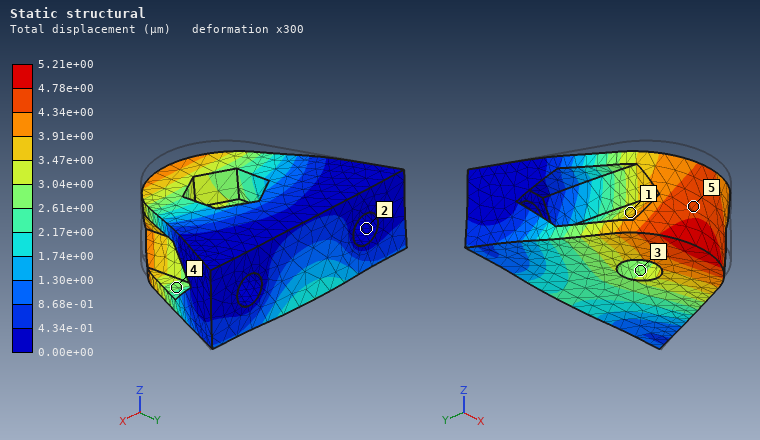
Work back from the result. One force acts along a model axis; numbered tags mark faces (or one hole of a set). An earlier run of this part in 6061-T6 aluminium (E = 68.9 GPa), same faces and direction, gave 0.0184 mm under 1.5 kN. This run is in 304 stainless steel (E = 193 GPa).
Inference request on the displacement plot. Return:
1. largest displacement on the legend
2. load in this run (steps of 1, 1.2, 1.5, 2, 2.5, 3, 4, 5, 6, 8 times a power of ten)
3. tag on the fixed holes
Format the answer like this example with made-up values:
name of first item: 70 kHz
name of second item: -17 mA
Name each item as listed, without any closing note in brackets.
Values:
largest displacement on the legend: 5.21e+00 µm
load in this run: 1.2 kN
tag on the fixed holes: 2
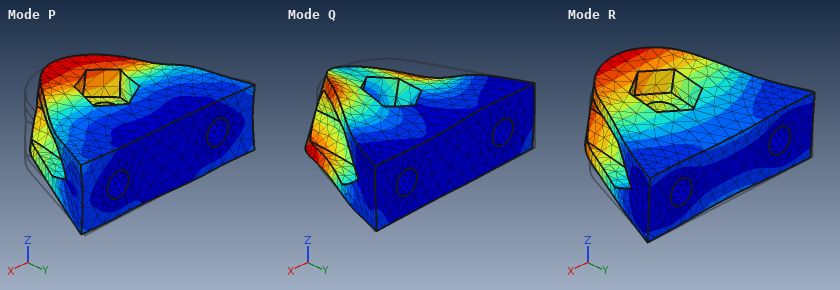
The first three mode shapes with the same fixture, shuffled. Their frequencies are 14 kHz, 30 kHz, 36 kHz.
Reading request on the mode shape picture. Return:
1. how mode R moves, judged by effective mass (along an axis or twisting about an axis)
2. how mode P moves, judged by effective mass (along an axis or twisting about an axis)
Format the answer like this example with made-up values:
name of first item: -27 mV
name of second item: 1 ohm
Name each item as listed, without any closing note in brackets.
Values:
how mode R moves, judged by effective mass: along Z
how mode P moves, judged by effective mass: along X
